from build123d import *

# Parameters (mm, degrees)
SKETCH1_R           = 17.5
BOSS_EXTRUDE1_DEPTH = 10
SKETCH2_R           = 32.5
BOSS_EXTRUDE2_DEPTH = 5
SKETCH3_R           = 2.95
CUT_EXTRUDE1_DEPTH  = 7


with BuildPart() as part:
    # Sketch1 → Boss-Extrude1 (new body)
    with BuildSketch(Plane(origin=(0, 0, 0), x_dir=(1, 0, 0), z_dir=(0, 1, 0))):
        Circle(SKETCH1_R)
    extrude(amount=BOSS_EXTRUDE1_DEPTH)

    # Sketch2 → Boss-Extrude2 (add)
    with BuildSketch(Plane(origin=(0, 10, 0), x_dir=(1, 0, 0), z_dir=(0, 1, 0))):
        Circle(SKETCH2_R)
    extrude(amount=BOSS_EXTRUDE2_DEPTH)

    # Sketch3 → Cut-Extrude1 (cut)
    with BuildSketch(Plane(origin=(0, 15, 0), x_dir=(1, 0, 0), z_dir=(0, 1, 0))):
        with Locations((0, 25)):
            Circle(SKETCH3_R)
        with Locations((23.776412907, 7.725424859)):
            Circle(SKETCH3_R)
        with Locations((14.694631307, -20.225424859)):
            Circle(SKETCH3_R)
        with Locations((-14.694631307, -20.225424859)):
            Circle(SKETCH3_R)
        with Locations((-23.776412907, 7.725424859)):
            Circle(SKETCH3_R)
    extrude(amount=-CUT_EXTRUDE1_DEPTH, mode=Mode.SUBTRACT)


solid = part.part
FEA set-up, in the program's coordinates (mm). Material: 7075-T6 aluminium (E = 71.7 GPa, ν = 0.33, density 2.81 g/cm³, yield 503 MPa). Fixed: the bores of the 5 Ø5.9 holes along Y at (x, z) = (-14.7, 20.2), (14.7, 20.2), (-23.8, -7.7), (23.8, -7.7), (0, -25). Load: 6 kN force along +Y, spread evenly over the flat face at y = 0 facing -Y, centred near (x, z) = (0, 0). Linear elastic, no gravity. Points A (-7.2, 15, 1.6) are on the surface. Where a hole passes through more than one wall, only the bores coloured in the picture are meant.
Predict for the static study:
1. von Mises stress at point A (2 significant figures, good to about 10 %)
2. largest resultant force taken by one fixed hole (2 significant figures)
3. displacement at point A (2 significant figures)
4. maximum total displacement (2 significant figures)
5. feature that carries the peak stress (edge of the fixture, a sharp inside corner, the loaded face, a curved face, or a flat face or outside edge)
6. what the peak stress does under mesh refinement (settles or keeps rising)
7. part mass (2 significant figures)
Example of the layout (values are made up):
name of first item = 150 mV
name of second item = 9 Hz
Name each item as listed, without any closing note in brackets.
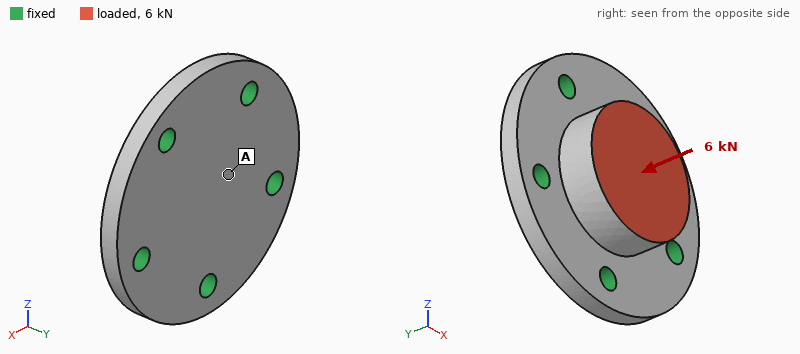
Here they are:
von Mises stress at point A = 10 MPa
largest resultant force taken by one fixed hole = 1.3 kN
displacement at point A = 12 µm
maximum total displacement = 12 µm
feature that carries the peak stress = edge of the fixture
what the peak stress does under mesh refinement = keeps rising
part mass = 72 g
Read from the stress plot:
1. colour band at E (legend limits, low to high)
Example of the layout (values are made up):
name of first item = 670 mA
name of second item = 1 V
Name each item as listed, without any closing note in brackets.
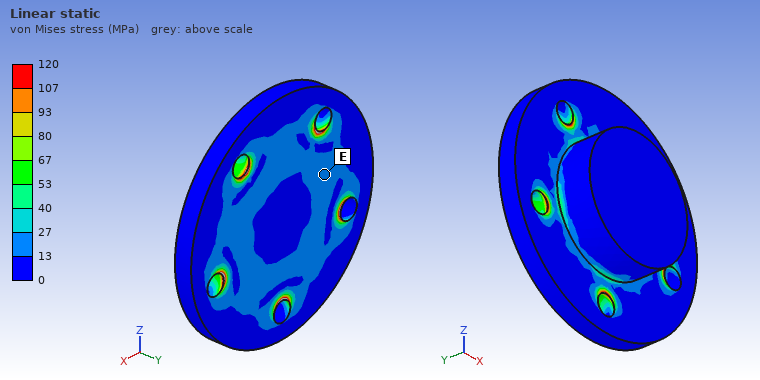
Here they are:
colour band at E = 13 to 27 MPa
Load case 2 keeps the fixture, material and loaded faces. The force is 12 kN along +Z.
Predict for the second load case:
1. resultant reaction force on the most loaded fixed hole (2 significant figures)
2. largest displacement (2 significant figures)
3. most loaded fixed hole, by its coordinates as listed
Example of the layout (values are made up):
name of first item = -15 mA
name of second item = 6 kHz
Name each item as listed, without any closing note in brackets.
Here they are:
resultant reaction force on the most loaded fixed hole = 4.4 kN
largest displacement = 32 µm
most loaded fixed hole, by its coordinates as listed = (0, -25)
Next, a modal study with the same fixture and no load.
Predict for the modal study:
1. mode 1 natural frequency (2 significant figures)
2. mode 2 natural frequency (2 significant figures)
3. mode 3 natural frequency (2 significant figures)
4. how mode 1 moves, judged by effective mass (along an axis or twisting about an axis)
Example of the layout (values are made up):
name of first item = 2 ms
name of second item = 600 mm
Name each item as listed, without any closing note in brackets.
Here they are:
mode 1 natural frequency = 18 kHz
mode 2 natural frequency = 22 kHz
mode 3 natural frequency = 22 kHz
how mode 1 moves, judged by effective mass = along Y
